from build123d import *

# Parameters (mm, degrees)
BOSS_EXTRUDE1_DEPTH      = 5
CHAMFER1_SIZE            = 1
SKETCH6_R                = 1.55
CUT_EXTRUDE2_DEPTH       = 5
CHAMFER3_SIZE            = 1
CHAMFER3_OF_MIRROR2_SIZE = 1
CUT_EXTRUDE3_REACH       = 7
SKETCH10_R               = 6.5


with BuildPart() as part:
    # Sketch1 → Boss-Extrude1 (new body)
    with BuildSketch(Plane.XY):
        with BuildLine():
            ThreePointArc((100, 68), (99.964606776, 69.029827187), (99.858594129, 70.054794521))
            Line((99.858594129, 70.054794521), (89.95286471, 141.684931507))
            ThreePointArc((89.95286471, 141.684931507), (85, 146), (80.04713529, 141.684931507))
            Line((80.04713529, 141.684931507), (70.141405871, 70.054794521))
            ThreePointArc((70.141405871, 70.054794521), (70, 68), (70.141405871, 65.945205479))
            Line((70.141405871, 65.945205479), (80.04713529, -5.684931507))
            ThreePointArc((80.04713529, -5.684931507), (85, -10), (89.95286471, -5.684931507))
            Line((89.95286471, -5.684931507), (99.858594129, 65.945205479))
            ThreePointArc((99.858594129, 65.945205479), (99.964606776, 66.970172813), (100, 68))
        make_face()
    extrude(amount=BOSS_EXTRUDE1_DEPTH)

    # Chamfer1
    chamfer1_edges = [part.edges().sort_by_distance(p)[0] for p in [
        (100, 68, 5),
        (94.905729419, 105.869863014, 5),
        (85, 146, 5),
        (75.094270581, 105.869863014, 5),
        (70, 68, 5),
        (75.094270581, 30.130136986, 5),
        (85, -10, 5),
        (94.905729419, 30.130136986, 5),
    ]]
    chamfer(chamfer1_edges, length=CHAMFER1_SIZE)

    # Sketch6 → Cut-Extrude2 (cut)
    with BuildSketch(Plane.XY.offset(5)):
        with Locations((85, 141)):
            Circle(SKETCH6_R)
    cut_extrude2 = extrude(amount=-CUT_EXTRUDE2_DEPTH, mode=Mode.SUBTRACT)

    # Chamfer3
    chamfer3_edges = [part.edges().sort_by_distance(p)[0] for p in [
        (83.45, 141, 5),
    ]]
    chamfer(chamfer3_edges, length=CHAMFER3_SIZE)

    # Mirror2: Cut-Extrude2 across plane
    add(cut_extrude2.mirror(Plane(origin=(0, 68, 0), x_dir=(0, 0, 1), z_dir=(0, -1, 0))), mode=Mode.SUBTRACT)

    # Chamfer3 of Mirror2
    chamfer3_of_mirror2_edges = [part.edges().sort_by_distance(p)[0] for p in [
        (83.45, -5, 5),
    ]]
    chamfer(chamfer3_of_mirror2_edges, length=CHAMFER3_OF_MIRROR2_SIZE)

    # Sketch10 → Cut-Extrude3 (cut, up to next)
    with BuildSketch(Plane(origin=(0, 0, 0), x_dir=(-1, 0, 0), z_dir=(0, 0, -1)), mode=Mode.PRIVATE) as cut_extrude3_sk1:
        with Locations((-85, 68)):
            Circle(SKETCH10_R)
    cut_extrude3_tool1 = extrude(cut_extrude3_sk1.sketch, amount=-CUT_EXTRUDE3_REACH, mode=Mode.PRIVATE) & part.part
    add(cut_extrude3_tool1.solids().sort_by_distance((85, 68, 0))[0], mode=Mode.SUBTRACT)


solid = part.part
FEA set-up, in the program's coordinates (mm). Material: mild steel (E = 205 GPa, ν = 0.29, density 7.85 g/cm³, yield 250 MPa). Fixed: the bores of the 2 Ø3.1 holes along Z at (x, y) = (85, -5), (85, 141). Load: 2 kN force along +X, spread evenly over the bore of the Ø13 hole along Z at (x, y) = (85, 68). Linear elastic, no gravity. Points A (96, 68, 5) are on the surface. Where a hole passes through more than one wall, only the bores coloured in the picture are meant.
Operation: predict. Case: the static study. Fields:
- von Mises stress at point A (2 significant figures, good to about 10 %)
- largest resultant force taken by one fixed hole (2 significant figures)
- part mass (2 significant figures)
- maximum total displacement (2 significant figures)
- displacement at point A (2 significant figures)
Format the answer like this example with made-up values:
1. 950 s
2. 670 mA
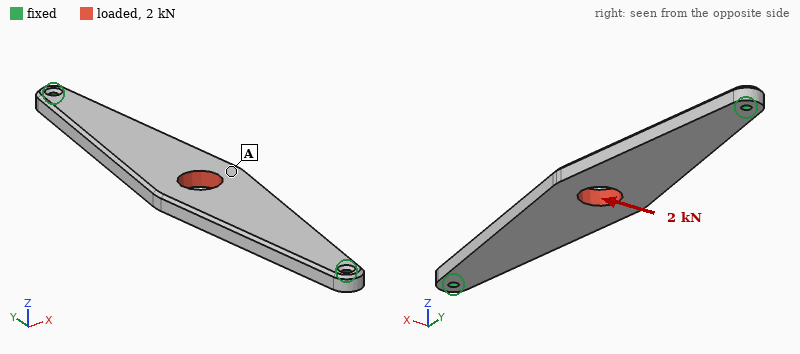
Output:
1. 62 MPa
2. 1.0 kN
3. 110 g
4. 85 µm
5. 84 µm
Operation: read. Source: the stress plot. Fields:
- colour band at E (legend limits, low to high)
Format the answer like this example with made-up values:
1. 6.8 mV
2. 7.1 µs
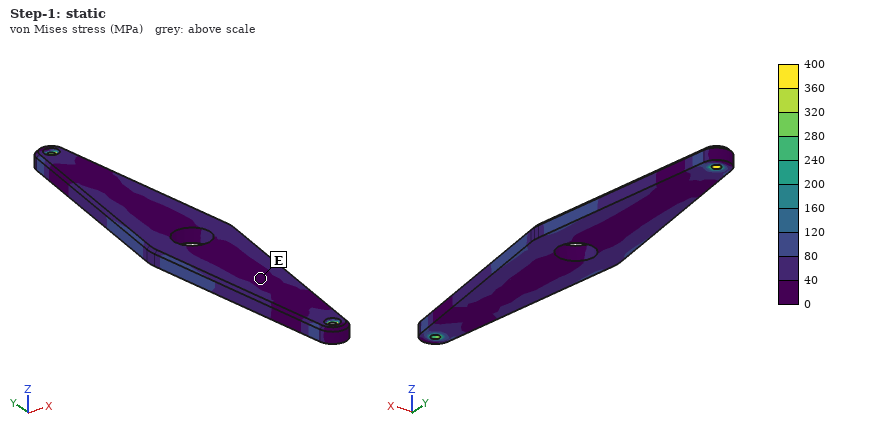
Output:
1. 0 to 40 MPa
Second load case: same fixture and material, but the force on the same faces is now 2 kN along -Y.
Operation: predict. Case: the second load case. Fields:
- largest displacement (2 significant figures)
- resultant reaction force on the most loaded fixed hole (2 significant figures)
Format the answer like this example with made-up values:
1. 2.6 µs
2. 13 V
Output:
1. 4.2 µm
2. 1.0 kN
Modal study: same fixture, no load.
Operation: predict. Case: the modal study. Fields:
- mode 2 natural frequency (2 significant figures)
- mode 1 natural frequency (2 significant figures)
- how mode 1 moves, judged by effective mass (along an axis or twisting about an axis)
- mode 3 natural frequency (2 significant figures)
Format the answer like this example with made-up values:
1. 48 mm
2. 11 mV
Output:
1. 3000 Hz
2. 980 Hz
3. along Z
4. 3000 Hz
